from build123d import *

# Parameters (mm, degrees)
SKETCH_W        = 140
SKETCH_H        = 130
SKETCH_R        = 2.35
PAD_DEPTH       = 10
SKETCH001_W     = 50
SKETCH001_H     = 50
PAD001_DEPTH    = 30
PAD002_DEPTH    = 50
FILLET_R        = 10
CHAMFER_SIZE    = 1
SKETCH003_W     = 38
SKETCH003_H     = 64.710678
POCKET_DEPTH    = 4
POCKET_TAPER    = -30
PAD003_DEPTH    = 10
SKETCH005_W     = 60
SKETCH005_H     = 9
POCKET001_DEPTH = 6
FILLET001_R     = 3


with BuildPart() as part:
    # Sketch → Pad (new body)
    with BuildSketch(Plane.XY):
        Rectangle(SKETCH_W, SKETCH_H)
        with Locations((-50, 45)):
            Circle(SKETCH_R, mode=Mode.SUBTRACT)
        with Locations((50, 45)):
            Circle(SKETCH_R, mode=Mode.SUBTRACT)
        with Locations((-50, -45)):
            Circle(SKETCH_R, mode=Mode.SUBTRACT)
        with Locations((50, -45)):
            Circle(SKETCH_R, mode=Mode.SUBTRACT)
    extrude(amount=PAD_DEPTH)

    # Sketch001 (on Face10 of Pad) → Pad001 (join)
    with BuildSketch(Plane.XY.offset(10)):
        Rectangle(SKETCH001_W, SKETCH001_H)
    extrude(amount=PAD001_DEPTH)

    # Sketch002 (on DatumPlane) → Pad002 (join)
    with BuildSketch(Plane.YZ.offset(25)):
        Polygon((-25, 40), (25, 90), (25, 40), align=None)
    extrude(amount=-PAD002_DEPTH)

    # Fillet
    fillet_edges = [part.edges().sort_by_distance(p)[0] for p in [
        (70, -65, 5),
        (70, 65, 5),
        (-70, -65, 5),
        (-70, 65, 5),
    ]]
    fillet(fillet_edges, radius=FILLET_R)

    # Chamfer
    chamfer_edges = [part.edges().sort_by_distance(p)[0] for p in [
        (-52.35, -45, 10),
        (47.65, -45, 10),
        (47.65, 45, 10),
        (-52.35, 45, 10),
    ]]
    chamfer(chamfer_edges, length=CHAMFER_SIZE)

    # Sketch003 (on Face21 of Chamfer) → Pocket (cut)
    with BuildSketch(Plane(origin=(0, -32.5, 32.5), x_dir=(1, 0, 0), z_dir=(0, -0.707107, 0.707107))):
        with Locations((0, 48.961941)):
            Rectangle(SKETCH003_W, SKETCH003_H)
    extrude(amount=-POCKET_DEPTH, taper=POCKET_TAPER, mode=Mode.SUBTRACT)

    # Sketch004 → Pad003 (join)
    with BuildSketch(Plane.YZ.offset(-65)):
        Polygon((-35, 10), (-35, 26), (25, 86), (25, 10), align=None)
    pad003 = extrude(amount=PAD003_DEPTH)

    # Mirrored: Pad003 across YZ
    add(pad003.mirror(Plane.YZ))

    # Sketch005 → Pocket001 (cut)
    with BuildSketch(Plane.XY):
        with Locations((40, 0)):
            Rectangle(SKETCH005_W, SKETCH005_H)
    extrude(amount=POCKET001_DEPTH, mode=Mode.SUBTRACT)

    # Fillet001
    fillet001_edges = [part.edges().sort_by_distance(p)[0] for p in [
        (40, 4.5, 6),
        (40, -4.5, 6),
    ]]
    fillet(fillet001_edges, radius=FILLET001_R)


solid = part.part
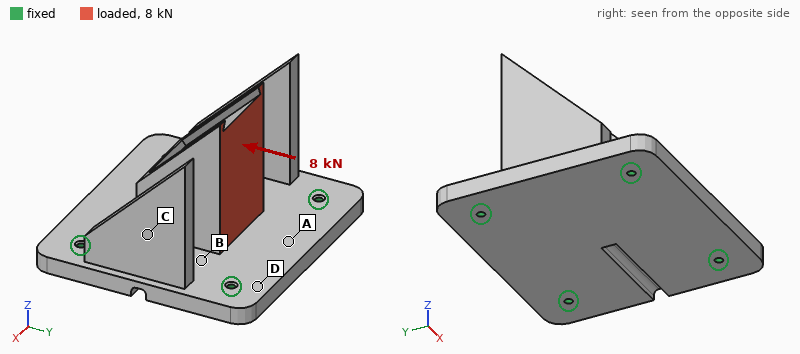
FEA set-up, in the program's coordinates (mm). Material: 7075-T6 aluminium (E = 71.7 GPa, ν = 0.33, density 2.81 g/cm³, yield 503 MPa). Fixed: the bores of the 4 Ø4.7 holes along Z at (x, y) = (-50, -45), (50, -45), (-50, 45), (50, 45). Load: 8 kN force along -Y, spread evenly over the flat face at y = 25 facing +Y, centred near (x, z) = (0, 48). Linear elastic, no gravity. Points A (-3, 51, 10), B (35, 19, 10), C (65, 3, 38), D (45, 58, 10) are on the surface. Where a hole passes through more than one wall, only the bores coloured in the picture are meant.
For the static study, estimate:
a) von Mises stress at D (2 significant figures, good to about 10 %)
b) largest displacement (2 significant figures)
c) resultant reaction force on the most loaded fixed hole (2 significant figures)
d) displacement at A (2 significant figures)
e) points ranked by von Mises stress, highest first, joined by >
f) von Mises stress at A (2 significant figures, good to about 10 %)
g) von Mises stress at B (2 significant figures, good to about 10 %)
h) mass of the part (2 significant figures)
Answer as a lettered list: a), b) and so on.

a) 15 MPa
b) 0.20 mm
c) 3.1 kN
d) 0.055 mm
e) B > A > D > C
f) 21 MPa
g) 31 MPa
h) 1.0 kg
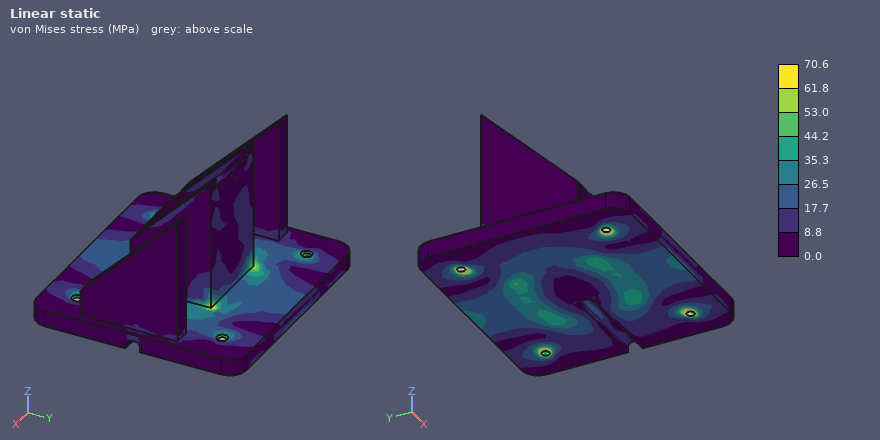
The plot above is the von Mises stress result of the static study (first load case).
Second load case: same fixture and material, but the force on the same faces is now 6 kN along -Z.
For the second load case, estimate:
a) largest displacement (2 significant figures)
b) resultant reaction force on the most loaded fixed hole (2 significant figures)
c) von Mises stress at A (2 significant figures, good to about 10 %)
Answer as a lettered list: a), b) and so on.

a) 0.12 mm
b) 2.6 kN
c) 23 MPa
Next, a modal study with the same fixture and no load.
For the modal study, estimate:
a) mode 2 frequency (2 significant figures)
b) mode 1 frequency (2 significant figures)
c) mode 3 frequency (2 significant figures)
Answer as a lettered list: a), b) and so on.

a) 1800 Hz
b) 1700 Hz
c) 2500 Hz
